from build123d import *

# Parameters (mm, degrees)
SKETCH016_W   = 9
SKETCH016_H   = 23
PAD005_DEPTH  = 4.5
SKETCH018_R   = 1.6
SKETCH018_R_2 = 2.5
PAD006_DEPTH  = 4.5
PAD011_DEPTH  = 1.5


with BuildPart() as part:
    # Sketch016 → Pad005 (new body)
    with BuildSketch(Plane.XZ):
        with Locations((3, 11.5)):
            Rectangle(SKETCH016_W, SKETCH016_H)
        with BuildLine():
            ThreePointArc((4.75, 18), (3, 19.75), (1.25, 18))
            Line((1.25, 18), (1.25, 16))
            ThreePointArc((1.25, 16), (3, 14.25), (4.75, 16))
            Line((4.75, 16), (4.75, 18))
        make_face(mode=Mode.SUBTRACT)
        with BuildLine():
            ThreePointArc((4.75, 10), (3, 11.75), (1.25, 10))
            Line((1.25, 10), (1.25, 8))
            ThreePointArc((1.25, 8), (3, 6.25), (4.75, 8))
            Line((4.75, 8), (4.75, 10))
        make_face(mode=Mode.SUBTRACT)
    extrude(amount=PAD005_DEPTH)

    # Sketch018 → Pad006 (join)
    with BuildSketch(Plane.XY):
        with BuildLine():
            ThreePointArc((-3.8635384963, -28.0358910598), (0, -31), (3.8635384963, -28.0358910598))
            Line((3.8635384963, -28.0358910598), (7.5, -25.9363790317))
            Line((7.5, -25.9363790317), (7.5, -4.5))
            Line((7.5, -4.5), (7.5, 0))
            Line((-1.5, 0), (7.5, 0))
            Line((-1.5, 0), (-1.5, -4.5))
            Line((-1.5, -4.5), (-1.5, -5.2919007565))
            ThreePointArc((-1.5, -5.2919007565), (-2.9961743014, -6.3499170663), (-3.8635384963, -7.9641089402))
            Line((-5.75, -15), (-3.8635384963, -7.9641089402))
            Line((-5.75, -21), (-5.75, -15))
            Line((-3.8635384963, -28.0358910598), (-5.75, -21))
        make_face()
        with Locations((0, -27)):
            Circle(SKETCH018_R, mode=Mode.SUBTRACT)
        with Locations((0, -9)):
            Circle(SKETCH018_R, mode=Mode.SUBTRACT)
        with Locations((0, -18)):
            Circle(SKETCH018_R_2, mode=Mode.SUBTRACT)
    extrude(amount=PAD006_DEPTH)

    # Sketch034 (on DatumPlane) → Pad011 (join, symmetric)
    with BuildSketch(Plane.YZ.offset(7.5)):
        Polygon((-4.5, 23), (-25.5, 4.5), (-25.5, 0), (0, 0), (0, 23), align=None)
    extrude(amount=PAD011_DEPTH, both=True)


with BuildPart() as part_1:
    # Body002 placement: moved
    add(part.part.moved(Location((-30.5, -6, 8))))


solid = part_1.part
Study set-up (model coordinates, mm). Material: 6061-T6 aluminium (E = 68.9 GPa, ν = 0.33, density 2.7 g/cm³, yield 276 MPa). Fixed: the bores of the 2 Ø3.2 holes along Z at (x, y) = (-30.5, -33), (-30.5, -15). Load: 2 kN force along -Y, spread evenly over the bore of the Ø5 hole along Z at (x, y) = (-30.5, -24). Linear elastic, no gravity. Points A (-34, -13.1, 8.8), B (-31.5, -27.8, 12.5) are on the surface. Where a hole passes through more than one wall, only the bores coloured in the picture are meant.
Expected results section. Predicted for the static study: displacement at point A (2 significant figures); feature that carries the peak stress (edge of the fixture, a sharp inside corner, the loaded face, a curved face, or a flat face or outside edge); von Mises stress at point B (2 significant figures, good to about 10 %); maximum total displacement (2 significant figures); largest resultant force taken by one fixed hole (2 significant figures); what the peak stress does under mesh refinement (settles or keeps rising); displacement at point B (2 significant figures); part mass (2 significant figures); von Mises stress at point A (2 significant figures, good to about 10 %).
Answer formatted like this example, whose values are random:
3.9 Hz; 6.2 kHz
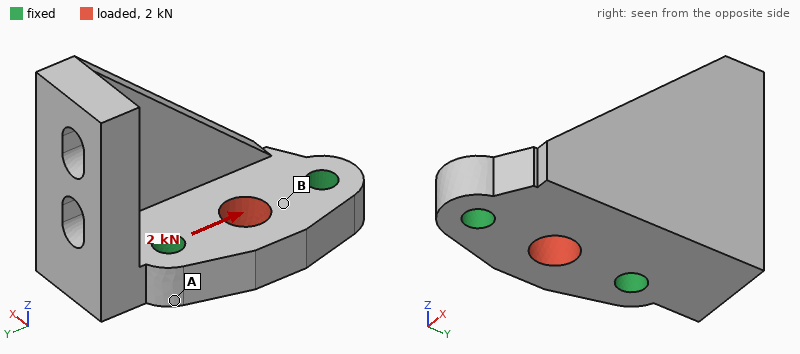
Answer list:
0.60 µm; edge of the fixture; 36 MPa; 3.5 µm; 1.0 kN; keeps rising; 2.1 µm; 7.7 g; 11 MPa
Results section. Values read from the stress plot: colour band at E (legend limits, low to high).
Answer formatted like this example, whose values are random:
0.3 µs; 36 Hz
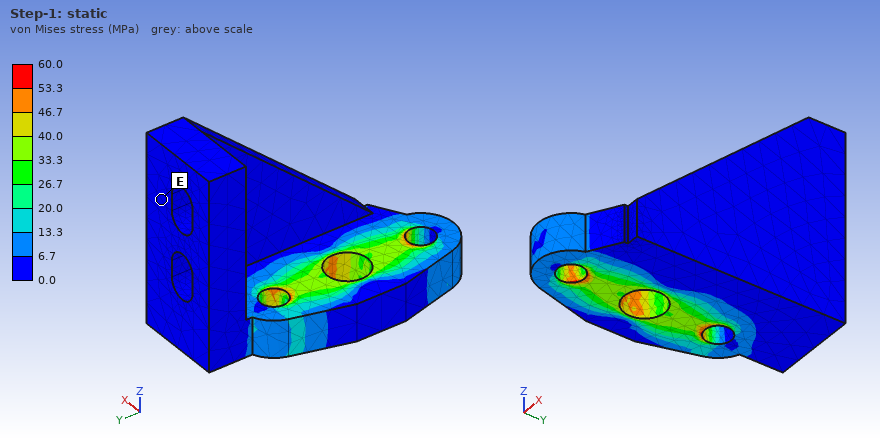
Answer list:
0.0 to 6.7 MPa
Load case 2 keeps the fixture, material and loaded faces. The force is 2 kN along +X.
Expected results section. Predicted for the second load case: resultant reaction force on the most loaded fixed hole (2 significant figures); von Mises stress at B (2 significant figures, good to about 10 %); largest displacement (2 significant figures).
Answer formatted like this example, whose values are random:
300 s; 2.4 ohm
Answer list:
1.0 kN; 38 MPa; 8.6 µm
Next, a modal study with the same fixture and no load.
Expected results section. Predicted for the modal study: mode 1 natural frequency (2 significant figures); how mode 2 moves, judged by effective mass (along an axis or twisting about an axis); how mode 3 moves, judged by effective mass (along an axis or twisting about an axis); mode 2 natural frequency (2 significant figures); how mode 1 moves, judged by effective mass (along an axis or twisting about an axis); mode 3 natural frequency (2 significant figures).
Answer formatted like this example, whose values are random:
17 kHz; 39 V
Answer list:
7300 Hz; along Y; along Z; 12 kHz; along X; 22 kHz
